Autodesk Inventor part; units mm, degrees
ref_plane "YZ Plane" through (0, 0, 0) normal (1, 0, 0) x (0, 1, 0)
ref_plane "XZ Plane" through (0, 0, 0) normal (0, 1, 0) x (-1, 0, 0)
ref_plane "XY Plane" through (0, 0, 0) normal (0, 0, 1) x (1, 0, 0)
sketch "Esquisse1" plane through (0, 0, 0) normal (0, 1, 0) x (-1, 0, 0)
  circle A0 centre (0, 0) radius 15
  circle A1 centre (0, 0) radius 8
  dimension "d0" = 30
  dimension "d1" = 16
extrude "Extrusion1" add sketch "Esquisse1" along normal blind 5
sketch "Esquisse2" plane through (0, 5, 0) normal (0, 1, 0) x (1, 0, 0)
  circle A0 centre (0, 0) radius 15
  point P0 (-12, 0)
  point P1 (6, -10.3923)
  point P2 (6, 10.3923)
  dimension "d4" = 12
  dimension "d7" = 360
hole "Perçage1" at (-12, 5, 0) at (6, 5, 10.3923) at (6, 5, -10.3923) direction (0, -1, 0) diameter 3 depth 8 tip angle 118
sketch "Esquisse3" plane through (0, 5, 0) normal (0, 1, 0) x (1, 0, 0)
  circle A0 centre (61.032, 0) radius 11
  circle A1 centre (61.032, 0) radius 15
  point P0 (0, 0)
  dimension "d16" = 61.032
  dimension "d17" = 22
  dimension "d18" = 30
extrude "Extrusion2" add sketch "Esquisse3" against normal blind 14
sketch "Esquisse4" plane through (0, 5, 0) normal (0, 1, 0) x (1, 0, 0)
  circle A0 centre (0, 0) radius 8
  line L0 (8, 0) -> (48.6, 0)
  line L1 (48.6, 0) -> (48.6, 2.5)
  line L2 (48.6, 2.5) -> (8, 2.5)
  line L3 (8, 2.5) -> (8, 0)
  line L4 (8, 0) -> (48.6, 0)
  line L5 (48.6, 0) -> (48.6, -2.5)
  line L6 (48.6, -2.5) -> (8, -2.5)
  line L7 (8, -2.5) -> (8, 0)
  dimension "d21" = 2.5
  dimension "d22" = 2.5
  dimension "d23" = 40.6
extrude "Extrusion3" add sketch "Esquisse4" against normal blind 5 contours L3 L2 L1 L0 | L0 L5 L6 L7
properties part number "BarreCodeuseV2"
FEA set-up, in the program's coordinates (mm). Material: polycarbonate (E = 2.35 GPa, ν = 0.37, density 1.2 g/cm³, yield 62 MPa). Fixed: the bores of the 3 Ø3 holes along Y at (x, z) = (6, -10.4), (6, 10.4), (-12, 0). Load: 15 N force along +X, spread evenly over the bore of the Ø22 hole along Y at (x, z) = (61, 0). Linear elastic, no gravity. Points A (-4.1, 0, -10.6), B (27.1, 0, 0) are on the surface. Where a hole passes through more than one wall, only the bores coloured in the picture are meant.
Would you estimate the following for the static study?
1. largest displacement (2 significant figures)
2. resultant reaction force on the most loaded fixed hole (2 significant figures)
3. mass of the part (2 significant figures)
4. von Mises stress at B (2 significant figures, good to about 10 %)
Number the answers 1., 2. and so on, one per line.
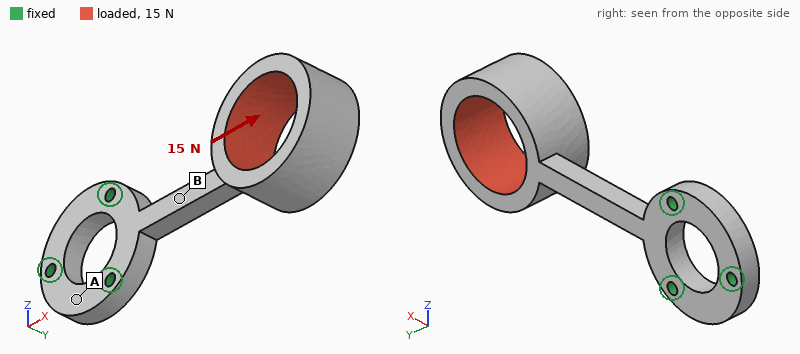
1. 1.1 mm
2. 9.8 N
3. 9.3 g
4. 3.8 MPa
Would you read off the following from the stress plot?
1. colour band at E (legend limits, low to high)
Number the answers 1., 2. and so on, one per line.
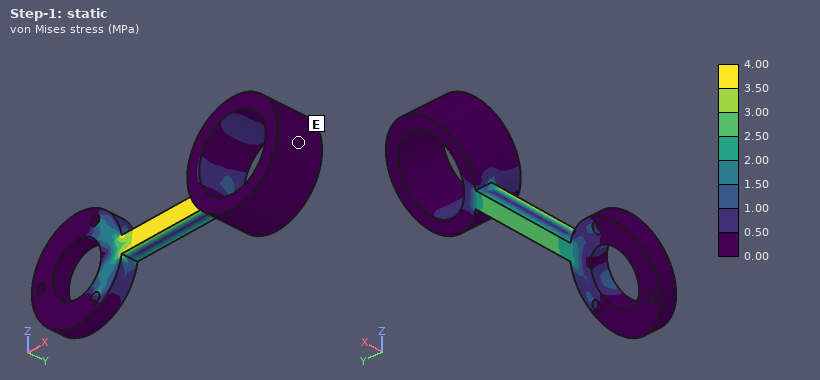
1. 0.00 to 0.50 MPa
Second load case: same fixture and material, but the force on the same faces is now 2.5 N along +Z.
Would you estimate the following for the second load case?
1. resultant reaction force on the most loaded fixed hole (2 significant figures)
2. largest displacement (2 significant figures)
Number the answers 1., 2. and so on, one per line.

1. 8.3 N
2. 1.1 mm
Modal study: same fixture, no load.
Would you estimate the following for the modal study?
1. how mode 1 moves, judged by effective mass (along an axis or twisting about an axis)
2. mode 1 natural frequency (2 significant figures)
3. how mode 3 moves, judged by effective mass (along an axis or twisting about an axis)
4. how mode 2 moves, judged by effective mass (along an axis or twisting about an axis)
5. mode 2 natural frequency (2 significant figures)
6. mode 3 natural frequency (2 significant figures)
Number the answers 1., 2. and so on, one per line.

1. along Y
2. 100 Hz
3. twisting about X
4. along Z
5. 110 Hz
6. 320 Hz
